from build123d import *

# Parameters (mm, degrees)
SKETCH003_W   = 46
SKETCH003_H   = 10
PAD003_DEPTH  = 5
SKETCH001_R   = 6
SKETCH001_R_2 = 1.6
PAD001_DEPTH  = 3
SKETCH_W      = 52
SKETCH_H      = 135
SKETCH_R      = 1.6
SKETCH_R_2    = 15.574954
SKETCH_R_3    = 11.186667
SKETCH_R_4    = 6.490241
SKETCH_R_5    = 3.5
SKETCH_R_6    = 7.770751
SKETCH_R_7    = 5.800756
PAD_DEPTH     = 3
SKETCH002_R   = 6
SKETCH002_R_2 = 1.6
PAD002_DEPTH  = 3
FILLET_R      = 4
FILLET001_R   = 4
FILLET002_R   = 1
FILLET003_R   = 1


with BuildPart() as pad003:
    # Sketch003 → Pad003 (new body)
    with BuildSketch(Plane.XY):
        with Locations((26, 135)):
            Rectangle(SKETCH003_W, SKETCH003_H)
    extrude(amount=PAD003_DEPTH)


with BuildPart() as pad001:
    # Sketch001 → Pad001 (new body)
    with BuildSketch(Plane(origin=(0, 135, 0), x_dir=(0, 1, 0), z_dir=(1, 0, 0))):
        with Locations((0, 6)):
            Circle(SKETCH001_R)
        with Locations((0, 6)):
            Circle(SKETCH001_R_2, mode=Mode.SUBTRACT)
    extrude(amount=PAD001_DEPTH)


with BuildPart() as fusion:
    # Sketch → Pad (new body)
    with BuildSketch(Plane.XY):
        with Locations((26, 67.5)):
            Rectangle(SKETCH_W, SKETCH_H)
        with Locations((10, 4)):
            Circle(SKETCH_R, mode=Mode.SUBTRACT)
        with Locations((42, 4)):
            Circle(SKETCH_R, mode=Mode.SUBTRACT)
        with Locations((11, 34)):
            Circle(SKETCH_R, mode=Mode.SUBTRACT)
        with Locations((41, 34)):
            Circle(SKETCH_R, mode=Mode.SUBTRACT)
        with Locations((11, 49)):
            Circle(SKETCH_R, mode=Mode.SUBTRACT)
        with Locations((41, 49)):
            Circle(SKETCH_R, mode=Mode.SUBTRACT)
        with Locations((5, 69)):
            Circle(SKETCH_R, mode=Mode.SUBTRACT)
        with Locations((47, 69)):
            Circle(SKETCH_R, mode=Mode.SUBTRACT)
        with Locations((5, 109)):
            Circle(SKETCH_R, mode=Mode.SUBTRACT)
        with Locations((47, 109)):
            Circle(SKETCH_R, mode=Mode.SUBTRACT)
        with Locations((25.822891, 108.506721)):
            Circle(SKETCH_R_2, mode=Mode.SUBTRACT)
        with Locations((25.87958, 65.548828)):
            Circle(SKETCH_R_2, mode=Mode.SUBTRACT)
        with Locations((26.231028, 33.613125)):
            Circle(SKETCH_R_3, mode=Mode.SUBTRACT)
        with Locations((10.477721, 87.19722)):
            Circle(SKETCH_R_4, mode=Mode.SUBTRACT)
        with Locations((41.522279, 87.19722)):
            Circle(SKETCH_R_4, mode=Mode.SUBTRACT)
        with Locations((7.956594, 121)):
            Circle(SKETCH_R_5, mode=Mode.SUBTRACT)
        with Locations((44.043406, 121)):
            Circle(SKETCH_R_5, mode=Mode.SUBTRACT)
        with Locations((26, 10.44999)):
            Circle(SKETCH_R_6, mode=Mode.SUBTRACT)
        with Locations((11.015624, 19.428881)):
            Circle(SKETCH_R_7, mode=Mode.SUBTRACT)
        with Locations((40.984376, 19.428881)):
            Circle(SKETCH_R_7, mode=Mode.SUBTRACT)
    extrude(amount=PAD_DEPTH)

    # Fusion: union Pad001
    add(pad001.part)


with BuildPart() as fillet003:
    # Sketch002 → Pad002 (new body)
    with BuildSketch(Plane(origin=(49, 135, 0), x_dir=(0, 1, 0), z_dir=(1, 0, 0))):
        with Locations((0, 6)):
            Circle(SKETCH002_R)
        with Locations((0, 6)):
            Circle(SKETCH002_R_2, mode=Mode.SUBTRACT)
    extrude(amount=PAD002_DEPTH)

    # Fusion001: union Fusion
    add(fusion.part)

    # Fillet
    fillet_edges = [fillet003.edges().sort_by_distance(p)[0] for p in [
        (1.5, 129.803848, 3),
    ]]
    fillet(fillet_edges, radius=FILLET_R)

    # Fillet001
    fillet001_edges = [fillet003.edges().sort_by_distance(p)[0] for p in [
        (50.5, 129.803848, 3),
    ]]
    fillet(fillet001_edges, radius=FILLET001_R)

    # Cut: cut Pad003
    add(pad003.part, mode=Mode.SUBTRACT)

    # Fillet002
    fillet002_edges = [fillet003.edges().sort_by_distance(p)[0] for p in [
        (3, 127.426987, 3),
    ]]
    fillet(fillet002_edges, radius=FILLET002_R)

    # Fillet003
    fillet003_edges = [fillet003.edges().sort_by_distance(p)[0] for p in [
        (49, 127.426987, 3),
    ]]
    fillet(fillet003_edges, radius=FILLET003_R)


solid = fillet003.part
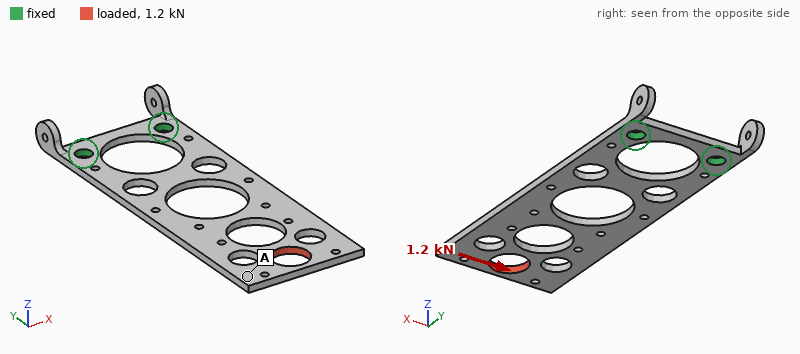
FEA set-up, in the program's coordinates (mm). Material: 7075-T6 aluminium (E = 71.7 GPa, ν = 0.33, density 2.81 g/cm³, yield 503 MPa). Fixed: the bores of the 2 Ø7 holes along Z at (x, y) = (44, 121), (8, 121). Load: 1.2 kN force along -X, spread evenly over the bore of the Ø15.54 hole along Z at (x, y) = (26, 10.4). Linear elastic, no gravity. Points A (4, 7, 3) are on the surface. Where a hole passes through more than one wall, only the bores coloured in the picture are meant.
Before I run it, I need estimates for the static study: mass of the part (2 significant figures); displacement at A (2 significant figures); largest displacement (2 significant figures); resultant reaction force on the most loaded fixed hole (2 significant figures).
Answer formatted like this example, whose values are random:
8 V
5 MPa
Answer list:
36 g
0.65 mm
0.69 mm
2.8 kN
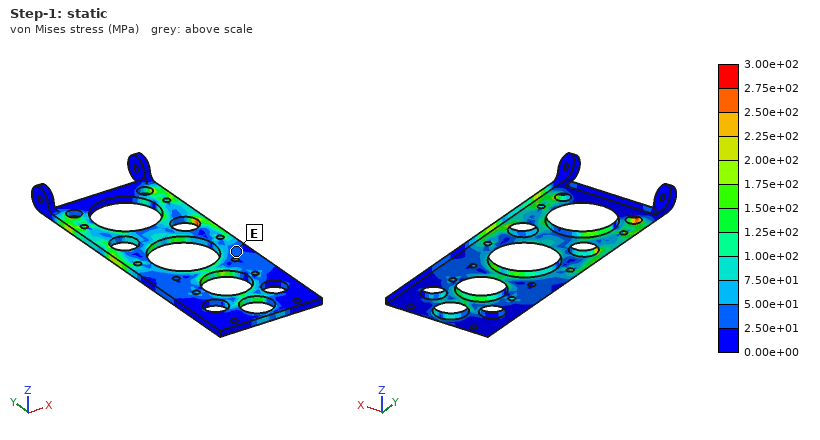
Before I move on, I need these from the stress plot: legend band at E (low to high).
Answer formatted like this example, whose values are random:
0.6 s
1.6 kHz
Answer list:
2.50e+01 to 5.00e+01 MPa
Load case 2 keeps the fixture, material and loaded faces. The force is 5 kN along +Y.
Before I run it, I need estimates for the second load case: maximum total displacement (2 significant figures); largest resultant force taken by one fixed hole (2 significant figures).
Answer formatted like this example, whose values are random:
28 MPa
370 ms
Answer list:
0.23 mm
2.5 kN
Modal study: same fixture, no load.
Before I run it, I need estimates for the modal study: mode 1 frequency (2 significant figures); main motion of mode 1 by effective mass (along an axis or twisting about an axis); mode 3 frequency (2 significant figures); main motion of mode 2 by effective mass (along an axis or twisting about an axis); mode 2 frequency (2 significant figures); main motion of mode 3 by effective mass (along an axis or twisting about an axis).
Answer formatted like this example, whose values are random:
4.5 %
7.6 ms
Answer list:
130 Hz
along Z
930 Hz
twisting about Y
620 Hz
along Z
